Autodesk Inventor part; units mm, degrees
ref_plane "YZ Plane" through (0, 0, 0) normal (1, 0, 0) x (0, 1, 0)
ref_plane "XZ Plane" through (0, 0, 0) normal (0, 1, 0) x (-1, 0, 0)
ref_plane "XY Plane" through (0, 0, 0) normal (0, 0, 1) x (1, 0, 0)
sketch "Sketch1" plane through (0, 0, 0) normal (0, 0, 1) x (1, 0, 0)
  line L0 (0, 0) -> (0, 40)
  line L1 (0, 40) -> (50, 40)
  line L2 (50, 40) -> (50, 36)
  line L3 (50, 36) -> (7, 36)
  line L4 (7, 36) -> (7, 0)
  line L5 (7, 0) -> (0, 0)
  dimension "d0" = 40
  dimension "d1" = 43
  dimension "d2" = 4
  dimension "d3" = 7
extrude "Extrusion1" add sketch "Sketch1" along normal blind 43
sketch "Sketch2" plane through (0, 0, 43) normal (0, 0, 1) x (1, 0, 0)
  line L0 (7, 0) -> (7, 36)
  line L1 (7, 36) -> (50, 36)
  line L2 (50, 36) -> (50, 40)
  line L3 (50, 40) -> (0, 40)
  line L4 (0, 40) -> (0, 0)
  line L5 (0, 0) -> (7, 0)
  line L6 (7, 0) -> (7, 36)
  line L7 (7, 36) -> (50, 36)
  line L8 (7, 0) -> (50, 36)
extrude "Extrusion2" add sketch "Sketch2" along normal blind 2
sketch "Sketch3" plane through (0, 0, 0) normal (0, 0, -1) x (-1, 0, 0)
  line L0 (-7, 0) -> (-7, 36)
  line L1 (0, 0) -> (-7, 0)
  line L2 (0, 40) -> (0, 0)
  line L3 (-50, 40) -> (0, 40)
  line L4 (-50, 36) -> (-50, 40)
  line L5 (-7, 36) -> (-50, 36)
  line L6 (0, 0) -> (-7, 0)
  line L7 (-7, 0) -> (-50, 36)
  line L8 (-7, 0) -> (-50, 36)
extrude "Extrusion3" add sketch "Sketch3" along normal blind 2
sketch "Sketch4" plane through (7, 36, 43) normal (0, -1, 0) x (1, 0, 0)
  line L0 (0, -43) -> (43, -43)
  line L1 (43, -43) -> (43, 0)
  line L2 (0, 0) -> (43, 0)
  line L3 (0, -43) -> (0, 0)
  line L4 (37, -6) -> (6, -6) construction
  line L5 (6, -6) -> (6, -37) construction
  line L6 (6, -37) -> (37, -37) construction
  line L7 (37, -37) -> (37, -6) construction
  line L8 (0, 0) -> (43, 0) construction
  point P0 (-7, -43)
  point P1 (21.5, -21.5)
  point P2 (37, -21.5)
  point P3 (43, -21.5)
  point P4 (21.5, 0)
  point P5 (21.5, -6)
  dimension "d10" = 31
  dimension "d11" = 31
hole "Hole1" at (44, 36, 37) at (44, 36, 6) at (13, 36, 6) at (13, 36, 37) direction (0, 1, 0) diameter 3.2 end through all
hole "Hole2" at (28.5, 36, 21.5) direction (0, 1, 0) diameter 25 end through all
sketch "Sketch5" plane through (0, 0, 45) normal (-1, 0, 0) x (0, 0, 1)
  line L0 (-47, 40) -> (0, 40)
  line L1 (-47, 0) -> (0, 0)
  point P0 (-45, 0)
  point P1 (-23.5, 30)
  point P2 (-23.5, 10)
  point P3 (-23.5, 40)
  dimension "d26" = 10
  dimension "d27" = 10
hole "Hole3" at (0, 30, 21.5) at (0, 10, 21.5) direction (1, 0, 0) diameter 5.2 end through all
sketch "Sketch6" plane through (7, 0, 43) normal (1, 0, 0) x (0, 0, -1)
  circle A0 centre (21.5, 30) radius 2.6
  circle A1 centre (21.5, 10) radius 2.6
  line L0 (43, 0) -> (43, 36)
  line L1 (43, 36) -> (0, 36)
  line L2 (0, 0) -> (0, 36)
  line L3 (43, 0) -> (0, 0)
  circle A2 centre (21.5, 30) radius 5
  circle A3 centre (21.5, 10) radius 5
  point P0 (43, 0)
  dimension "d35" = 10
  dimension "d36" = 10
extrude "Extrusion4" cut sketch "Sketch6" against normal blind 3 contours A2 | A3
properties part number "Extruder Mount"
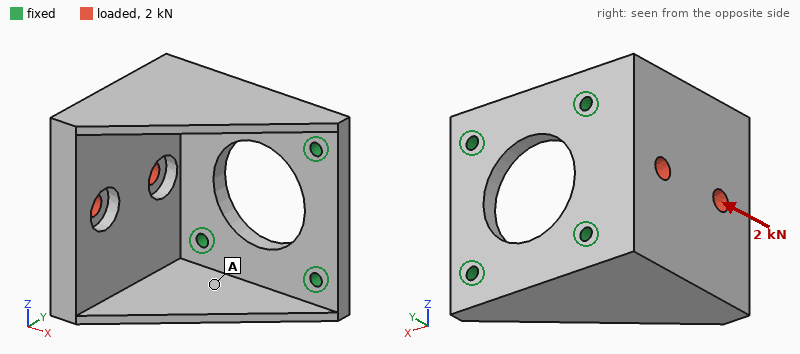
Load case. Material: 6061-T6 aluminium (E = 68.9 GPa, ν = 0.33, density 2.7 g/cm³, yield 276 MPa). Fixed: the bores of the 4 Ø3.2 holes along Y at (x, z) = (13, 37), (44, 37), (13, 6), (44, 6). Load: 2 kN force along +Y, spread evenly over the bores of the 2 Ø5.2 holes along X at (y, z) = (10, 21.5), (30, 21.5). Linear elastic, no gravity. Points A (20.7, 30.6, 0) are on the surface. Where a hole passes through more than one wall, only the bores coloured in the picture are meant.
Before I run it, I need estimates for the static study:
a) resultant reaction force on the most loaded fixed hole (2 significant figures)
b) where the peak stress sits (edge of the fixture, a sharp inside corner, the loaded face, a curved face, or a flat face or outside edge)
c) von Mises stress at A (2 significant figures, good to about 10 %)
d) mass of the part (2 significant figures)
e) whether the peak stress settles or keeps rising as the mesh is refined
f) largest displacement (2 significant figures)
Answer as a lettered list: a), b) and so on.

a) 1.3 kN
b) edge of the fixture
c) 13 MPa
d) 58 g
e) keeps rising
f) 53 µm
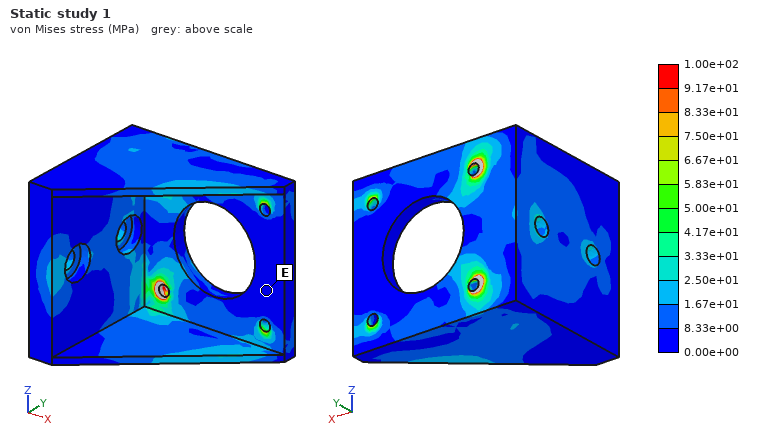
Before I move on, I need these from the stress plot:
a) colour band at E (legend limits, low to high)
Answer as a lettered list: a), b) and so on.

a) 0.00e+00 to 8.33e+00 MPa
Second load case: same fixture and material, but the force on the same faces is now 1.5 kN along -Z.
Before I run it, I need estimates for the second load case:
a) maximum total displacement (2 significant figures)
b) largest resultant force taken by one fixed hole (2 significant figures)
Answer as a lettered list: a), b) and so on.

a) 42 µm
b) 1.2 kN
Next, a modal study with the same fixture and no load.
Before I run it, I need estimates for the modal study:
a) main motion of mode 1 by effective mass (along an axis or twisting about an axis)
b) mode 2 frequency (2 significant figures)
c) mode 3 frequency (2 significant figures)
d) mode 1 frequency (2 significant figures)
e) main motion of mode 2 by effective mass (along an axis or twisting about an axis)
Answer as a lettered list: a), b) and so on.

a) along X
b) 5200 Hz
c) 7700 Hz
d) 4700 Hz
e) along Z
